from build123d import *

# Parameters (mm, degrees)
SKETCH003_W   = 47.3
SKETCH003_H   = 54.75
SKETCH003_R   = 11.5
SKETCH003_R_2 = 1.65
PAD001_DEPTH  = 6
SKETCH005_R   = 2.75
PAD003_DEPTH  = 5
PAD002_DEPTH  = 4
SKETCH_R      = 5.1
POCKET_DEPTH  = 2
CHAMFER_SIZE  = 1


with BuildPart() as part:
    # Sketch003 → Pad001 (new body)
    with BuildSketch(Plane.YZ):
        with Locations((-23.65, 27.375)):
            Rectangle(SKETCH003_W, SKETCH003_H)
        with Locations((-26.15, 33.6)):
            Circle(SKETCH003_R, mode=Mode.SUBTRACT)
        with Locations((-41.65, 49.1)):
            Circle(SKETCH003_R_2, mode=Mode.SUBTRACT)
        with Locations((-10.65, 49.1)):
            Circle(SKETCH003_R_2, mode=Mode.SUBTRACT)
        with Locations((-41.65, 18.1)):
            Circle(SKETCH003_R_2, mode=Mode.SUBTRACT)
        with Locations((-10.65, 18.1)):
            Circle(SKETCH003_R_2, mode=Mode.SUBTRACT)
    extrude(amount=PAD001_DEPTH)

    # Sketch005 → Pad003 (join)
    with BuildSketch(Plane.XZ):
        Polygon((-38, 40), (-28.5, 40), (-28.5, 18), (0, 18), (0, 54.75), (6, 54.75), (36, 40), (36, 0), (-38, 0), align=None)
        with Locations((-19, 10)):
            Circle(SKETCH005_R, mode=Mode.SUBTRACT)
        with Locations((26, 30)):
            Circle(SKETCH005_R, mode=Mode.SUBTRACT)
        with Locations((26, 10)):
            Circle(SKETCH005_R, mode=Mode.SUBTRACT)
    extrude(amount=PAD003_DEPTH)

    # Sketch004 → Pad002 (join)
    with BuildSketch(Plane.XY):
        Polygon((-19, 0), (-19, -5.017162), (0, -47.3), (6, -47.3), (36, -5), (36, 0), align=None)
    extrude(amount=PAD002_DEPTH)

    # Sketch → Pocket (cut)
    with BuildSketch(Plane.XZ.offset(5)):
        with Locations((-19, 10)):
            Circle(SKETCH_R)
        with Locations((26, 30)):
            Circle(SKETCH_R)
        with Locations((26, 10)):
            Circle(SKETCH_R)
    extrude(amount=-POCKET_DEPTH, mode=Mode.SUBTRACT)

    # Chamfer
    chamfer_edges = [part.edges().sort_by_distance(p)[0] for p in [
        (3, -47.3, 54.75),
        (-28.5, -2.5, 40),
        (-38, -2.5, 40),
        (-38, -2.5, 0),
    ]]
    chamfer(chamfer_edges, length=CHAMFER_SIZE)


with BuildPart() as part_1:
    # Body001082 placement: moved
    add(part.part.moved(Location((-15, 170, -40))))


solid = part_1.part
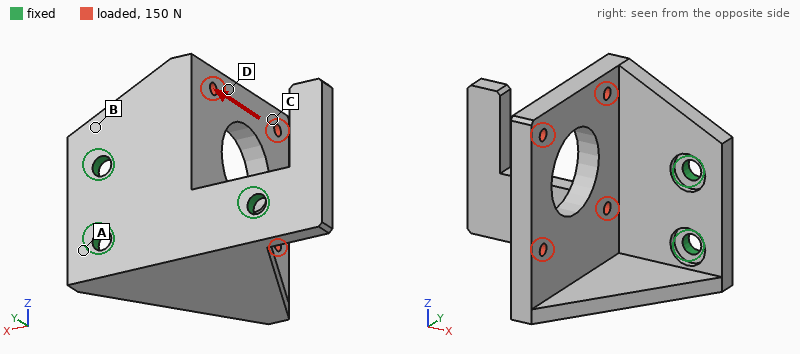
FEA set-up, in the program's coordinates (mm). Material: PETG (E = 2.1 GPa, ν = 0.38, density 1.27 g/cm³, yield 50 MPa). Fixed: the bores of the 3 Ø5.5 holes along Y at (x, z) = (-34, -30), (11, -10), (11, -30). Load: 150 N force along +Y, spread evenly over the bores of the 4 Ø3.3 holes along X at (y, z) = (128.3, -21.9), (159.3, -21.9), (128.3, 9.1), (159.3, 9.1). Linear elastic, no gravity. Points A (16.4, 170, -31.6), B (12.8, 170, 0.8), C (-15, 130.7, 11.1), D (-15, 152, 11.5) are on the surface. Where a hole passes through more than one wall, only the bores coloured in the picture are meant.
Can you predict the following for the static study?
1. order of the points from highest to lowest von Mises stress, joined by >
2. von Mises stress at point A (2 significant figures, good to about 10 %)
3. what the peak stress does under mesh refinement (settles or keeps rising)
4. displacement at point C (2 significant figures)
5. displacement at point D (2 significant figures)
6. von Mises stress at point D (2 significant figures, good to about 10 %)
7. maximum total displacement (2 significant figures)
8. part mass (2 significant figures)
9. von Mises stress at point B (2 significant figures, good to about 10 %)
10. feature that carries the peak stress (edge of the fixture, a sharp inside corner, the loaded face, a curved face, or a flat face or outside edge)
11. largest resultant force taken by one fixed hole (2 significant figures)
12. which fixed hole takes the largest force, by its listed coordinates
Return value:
B > A > D > C
4.3 MPa
keeps rising
1.1 mm
0.86 mm
2.9 MPa
1.2 mm
35 g
6.0 MPa
edge of the fixture
140 N
(11, -10)
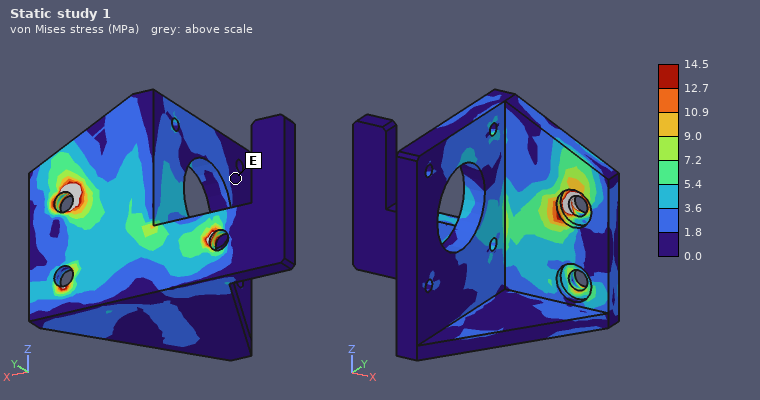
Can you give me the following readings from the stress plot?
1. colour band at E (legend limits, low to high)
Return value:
0.0 to 1.8 MPa
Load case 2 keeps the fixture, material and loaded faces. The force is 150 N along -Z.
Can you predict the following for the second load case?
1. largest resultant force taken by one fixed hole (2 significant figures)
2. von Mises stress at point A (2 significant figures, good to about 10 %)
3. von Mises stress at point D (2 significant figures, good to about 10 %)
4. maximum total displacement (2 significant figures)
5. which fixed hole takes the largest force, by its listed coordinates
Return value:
190 N
5.7 MPa
2.0 MPa
1.0 mm
(11, -10)
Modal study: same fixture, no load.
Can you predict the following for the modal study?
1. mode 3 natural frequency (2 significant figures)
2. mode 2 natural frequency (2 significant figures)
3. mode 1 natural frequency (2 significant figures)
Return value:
870 Hz
730 Hz
470 Hz
